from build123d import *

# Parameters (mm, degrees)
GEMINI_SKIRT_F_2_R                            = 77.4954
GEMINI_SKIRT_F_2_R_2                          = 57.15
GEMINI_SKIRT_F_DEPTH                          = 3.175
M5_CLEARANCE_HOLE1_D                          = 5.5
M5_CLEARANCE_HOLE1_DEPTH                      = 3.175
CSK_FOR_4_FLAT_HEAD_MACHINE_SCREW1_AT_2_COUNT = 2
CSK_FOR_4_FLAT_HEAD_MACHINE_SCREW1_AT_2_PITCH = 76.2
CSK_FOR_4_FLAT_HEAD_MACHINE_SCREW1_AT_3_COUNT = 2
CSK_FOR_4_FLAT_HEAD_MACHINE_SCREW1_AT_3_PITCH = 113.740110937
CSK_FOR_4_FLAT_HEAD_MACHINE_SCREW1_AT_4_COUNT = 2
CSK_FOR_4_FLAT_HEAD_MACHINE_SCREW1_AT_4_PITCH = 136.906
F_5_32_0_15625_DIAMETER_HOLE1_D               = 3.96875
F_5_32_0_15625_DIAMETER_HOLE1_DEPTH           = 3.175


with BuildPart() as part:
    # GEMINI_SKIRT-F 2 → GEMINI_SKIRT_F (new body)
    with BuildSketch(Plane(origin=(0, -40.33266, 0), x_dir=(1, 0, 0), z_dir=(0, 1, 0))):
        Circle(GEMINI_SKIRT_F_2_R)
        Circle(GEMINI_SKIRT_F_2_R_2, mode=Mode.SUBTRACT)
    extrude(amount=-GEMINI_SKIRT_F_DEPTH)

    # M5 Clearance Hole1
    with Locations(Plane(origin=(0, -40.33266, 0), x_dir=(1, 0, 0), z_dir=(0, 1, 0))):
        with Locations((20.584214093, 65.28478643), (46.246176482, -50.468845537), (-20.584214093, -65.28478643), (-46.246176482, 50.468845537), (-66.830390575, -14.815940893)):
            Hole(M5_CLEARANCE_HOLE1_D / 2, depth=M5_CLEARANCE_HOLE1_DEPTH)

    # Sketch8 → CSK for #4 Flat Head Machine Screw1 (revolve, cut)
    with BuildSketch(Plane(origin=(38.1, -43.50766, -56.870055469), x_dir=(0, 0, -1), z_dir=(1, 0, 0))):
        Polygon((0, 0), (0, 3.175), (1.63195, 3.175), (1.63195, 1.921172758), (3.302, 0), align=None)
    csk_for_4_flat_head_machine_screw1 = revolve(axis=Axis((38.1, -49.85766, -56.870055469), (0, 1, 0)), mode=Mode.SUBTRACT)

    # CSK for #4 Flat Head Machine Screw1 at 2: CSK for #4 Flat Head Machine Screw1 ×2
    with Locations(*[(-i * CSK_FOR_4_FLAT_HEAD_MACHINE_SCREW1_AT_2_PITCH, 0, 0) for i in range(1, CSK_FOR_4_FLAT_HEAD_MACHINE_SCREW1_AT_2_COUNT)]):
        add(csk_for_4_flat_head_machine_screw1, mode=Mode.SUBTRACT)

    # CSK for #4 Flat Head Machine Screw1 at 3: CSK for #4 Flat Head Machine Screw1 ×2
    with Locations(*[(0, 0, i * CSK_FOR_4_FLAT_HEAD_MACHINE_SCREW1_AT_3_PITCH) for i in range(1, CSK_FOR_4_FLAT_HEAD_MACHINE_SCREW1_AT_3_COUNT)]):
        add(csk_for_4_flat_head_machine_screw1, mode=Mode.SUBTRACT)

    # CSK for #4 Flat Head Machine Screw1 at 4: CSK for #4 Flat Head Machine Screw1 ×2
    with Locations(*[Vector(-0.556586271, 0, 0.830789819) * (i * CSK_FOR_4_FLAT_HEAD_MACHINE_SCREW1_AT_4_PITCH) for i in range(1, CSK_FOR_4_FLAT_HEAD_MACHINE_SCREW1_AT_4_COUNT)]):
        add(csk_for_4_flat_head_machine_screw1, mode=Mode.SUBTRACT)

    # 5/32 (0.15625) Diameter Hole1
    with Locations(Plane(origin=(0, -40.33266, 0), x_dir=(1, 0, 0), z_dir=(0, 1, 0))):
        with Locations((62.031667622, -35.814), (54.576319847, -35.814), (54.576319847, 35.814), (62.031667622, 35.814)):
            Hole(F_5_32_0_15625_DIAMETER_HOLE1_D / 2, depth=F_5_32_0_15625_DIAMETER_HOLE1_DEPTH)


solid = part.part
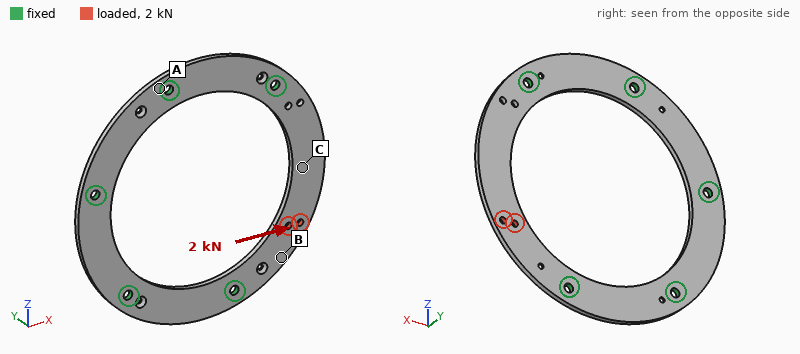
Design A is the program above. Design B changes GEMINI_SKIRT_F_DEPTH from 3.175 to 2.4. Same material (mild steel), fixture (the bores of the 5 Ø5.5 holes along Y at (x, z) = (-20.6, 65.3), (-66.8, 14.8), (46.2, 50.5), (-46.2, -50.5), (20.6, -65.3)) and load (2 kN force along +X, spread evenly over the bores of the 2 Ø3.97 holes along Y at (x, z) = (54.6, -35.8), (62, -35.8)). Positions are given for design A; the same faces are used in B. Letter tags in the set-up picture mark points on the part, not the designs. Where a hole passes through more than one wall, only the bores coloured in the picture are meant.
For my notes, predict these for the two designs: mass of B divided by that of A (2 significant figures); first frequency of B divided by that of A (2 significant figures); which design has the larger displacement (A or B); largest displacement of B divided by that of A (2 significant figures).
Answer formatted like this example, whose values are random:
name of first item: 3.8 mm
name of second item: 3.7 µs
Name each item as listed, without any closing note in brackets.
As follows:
mass of B divided by that of A: 0.76
first frequency of B divided by that of A: 0.76
which design has the larger displacement: B
largest displacement of B divided by that of A: 1.3
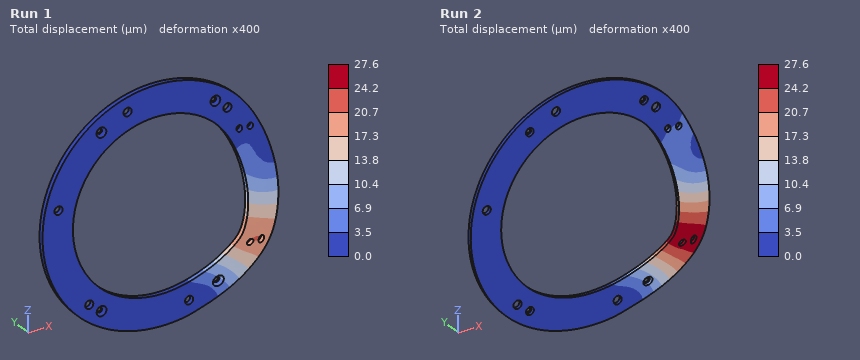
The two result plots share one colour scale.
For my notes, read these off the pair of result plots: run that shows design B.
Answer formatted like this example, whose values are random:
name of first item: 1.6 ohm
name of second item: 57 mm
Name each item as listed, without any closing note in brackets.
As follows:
run that shows design B: Run 2
